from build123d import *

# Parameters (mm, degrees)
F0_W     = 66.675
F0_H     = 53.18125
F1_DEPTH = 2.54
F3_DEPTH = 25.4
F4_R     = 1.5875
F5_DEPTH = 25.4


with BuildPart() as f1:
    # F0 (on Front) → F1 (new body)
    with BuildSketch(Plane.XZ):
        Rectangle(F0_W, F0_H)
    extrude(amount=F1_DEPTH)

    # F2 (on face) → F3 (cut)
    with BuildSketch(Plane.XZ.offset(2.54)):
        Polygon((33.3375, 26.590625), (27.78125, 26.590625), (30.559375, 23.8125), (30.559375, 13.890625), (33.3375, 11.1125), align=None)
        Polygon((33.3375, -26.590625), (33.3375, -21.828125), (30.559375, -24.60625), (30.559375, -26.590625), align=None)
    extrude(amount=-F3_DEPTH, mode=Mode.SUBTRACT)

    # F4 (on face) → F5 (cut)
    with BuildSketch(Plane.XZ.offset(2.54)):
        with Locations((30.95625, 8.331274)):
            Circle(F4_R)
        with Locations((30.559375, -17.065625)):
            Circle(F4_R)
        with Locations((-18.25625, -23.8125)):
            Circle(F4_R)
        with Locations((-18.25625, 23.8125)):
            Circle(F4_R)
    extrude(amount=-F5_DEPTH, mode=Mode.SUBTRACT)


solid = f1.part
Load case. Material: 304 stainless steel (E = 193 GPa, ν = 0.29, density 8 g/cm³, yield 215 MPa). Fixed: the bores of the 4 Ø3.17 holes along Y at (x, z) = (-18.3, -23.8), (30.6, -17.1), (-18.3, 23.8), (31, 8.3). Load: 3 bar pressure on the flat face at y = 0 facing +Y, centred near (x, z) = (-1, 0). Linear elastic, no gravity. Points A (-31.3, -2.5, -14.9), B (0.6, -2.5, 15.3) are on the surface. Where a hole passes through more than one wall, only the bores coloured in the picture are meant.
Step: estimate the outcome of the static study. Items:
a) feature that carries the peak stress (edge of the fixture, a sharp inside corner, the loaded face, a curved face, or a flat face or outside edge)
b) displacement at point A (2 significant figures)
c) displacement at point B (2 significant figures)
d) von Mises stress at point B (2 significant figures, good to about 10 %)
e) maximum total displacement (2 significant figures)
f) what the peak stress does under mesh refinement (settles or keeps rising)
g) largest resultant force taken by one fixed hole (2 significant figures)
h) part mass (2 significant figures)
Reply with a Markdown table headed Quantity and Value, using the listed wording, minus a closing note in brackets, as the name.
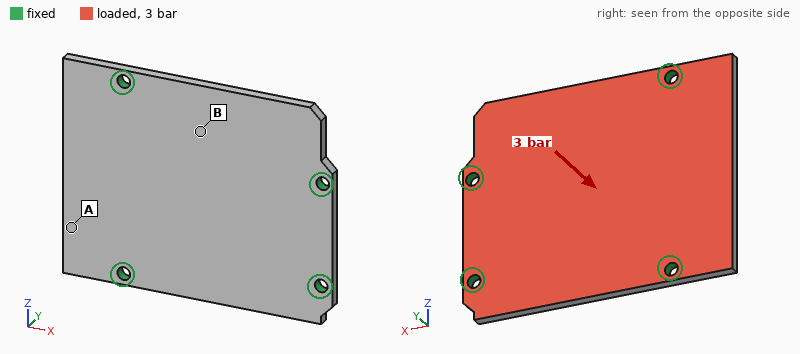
| Quantity | Value |
|---|---|
| feature that carries the peak stress | edge of the fixture |
| displacement at point A | 14 µm |
| displacement at point B | 27 µm |
| von Mises stress at point B | 33 MPa |
| maximum total displacement | 31 µm |
| what the peak stress does under mesh refinement | keeps rising |
| largest resultant force taken by one fixed hole | 320 N |
| part mass | 70 g |
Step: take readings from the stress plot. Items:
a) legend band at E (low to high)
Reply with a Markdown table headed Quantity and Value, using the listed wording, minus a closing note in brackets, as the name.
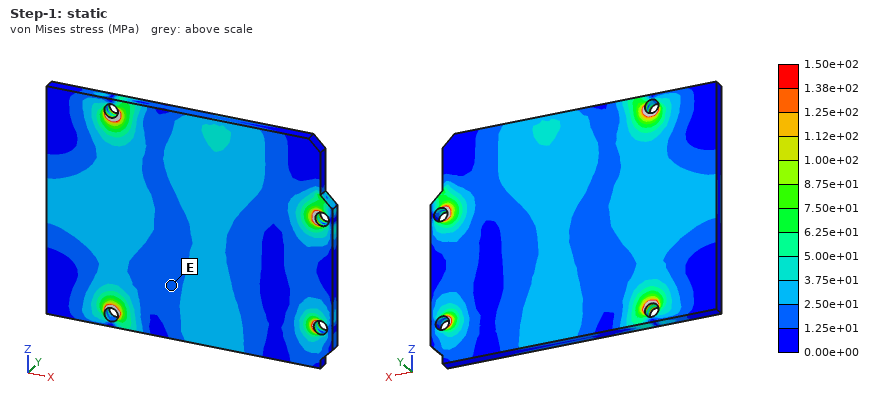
| Quantity | Value |
|---|---|
| legend band at E | 1.25e+01 to 2.50e+01 MPa |
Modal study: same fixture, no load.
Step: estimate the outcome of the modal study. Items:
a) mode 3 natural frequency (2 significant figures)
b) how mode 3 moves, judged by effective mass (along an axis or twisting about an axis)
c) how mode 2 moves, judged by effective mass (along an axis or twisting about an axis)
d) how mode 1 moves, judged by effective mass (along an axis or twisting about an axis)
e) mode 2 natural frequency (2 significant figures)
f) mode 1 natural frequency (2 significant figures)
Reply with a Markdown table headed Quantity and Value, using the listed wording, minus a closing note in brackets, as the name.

| Quantity | Value |
|---|---|
| mode 3 natural frequency | 5000 Hz |
| how mode 3 moves, judged by effective mass | twisting about X |
| how mode 2 moves, judged by effective mass | along Y |
| how mode 1 moves, judged by effective mass | along Y |
| mode 2 natural frequency | 4500 Hz |
| mode 1 natural frequency | 4000 Hz |
